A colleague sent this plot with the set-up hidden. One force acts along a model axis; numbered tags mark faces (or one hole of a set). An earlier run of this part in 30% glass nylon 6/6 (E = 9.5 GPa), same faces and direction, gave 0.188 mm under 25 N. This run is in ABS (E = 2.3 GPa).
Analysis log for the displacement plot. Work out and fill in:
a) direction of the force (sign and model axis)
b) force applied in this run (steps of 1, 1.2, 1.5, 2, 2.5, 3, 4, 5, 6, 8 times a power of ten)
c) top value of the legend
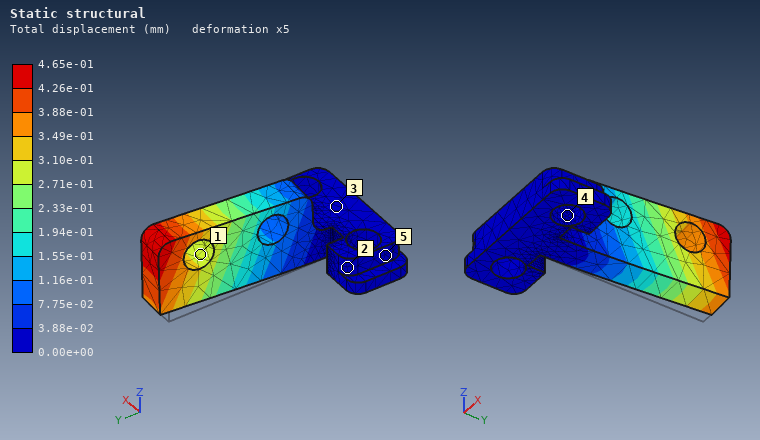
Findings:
+X
15 N
4.65e-01 mm
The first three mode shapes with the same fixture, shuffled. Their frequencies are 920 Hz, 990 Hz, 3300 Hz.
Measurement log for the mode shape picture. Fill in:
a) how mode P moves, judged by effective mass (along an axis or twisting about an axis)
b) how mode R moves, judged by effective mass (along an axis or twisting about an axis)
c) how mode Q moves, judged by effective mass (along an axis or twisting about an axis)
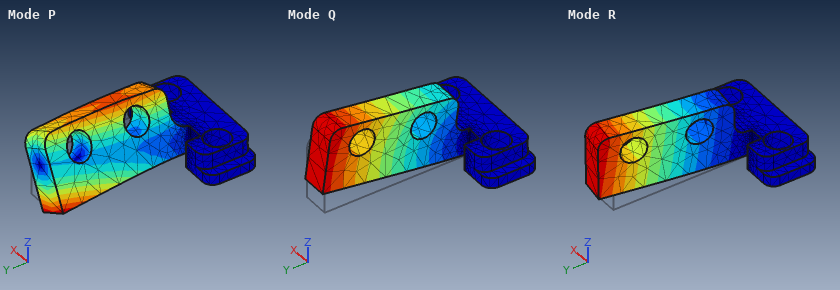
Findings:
twisting about Y
along X
along Z
